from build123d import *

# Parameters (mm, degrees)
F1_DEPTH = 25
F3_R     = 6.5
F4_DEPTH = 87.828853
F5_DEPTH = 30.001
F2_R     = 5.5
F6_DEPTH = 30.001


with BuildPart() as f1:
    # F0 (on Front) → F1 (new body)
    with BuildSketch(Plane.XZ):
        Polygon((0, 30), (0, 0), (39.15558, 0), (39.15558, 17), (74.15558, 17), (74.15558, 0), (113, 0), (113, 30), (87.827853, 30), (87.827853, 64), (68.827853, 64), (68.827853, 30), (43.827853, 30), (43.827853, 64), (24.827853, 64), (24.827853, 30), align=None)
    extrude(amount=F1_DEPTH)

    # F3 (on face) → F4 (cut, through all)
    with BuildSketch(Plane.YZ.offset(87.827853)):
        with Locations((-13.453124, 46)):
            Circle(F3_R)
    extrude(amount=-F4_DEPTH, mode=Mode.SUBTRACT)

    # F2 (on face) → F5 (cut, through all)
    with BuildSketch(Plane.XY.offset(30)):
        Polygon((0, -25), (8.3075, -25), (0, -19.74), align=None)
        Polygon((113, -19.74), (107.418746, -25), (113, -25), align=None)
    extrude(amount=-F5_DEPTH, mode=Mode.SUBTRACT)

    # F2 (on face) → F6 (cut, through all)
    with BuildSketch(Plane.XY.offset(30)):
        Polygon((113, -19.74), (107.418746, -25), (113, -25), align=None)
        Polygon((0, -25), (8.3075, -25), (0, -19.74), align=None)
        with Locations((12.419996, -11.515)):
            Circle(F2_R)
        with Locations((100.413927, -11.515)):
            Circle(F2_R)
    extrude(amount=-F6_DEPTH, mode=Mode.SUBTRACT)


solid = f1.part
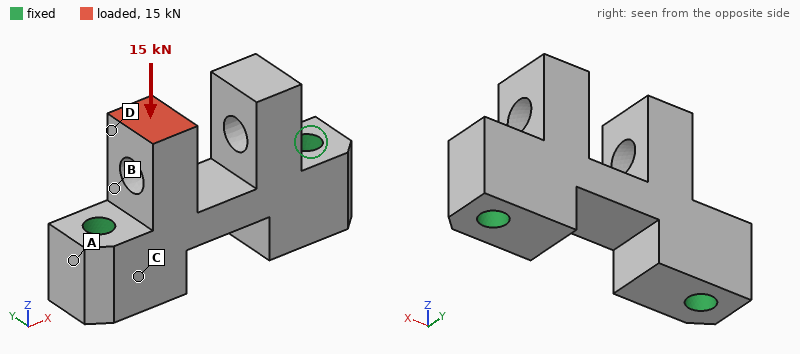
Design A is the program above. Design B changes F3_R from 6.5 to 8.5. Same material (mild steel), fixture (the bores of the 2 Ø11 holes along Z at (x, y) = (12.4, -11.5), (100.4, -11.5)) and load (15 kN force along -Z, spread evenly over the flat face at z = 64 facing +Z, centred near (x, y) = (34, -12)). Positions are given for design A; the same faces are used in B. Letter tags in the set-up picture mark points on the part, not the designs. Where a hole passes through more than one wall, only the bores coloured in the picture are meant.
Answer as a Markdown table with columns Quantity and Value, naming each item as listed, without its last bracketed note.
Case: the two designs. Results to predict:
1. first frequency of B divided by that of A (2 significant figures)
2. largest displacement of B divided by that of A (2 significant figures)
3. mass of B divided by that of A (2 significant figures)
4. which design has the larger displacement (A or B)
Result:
| Quantity | Value |
|---|---|
| first frequency of B divided by that of A | 0.95 |
| largest displacement of B divided by that of A | 1.3 |
| mass of B divided by that of A | 0.96 |
| which design has the larger displacement | B |
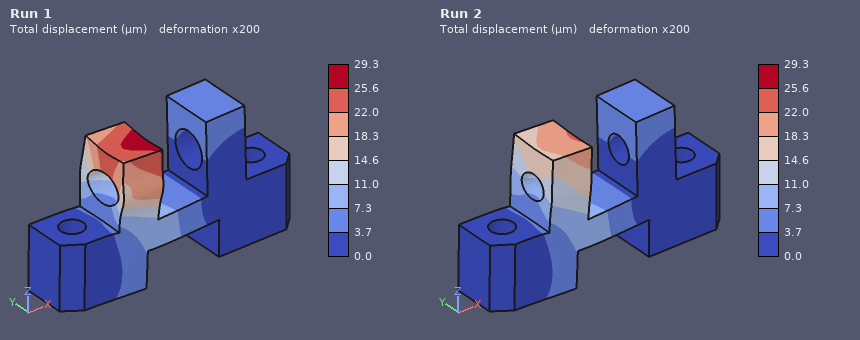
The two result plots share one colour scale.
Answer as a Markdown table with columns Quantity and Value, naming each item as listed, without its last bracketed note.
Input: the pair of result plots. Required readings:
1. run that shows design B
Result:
| Quantity | Value |
|---|---|
| run that shows design B | Run 1 |
